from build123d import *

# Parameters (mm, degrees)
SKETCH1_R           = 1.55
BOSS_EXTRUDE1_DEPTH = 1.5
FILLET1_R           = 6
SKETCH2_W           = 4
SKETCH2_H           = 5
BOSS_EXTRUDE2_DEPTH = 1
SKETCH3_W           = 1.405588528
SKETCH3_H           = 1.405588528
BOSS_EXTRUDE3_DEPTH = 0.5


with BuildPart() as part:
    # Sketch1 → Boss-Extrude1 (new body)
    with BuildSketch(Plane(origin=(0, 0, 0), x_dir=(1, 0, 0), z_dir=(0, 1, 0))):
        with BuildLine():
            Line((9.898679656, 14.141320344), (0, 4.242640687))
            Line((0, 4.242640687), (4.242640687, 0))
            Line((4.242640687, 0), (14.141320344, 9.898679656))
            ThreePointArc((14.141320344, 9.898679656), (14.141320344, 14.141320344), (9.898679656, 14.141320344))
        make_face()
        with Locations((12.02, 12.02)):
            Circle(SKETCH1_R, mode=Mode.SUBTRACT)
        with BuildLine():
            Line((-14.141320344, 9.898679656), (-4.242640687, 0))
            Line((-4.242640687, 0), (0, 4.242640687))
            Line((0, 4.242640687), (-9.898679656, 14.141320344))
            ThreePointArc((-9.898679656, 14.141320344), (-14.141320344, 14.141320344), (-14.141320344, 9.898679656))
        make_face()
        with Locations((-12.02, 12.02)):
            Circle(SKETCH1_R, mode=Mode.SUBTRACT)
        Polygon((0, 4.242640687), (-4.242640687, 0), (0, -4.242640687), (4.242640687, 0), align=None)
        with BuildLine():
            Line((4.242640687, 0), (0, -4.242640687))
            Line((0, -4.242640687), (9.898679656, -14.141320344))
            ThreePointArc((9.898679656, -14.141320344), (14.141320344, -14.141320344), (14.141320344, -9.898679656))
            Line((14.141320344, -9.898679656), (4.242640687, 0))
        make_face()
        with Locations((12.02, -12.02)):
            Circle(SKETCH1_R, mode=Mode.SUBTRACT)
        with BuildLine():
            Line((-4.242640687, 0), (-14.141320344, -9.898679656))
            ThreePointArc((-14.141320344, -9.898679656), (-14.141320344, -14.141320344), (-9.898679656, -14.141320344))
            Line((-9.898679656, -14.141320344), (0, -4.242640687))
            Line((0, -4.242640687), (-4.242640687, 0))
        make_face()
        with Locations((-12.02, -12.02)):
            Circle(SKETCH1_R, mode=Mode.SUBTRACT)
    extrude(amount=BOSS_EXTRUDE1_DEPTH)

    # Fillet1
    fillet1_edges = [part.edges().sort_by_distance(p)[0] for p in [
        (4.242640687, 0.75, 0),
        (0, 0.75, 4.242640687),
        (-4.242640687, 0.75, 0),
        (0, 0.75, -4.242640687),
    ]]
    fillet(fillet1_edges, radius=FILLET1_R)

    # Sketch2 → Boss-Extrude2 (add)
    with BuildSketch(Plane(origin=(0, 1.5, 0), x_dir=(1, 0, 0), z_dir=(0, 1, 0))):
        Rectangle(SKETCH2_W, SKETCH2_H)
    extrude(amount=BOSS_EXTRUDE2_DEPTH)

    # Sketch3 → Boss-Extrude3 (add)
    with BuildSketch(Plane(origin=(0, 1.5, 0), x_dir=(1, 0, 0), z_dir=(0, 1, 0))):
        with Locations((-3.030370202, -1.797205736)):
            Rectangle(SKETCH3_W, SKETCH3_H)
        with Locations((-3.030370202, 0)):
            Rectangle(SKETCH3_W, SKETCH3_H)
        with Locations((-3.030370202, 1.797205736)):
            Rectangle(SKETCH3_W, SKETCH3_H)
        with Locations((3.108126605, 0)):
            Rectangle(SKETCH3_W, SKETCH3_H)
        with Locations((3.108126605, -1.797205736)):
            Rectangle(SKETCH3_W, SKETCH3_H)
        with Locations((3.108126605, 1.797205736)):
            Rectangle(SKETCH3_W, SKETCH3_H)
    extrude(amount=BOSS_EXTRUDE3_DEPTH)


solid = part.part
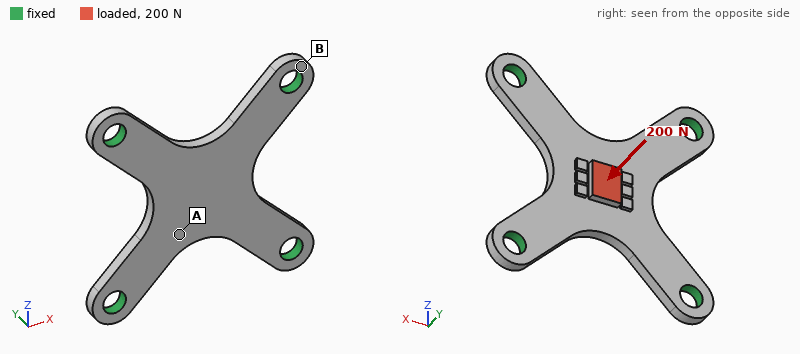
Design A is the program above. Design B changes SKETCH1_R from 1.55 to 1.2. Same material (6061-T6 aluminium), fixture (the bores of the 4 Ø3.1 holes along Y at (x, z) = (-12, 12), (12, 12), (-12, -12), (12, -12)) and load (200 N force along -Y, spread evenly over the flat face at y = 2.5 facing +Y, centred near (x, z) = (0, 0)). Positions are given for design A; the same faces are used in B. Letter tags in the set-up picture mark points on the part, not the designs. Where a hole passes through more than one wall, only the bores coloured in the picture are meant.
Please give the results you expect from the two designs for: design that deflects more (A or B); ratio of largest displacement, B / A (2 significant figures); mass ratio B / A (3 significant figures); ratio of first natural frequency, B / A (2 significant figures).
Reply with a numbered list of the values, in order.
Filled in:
1. B
2. 1.1
3. 1.03
4. 0.94
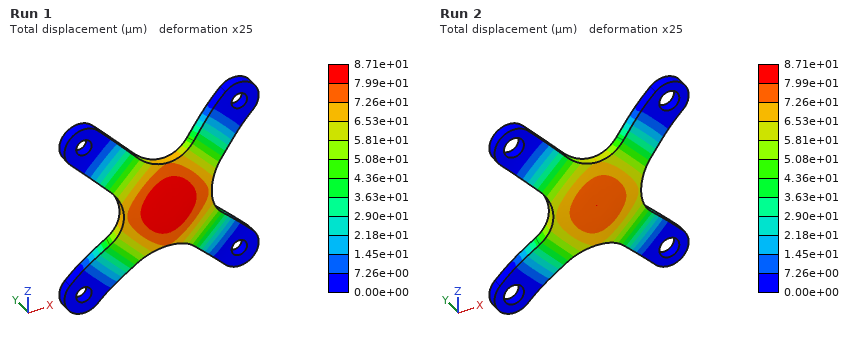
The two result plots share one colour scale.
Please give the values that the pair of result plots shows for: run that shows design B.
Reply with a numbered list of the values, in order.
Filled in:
1. Run 1
